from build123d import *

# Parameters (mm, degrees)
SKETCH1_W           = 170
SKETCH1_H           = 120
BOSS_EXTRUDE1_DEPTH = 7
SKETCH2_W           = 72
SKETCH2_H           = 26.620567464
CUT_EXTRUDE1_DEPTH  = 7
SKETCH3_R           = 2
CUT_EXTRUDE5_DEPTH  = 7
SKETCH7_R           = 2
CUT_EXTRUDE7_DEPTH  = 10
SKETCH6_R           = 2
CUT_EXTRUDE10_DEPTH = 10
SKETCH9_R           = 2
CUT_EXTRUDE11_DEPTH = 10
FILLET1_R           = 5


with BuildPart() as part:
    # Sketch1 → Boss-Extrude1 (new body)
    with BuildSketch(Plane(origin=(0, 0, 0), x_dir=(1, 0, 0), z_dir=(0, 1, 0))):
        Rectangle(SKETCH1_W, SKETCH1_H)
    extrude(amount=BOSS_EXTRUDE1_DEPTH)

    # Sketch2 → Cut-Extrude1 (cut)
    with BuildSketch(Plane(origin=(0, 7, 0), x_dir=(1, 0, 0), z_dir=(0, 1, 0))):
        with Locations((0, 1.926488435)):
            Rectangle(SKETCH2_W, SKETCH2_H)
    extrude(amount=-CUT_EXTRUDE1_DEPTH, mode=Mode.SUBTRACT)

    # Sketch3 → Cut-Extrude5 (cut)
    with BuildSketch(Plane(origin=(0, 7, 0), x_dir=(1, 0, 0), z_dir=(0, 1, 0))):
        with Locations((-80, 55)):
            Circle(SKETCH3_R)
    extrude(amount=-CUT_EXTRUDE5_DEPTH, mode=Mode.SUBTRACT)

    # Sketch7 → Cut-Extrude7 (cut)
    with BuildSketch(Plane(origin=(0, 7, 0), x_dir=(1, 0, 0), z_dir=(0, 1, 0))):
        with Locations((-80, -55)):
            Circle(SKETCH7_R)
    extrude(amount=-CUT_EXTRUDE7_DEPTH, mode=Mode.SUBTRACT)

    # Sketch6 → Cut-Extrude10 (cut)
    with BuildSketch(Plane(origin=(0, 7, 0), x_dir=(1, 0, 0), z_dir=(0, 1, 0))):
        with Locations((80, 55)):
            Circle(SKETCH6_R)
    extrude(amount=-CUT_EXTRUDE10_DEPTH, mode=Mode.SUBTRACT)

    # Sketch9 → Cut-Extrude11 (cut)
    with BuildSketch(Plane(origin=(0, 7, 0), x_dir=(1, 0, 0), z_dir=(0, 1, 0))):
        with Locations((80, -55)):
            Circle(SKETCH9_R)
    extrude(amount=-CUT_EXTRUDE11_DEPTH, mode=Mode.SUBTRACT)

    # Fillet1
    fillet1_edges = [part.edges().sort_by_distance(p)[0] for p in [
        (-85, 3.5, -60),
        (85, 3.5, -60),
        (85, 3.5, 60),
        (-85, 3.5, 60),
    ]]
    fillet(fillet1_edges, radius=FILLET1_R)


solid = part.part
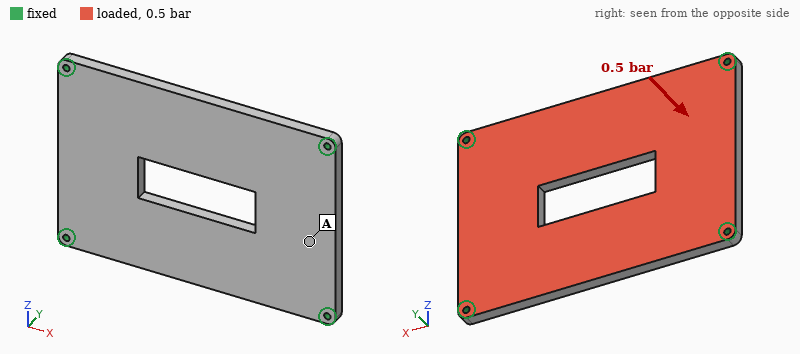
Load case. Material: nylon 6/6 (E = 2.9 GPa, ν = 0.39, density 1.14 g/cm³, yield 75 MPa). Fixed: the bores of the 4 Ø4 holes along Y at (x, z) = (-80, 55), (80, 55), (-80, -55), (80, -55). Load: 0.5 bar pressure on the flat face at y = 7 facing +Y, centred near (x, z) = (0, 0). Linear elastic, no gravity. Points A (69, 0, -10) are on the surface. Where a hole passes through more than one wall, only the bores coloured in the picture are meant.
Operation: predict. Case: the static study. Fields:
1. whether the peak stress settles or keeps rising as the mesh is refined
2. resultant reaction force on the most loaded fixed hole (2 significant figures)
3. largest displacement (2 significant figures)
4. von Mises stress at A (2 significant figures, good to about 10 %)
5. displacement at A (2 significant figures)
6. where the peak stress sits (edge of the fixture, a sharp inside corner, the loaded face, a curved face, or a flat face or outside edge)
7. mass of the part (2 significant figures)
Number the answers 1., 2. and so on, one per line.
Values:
1. keeps rising
2. 230 N
3. 2.5 mm
4. 5.6 MPa
5. 0.81 mm
6. edge of the fixture
7. 150 g
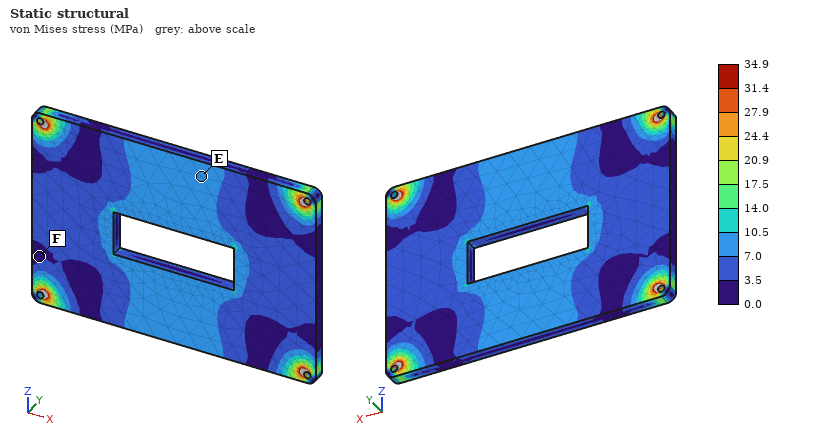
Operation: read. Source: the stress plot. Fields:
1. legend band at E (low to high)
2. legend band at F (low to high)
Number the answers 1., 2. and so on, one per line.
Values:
1. 7.0 to 10.5 MPa
2. 0.0 to 3.5 MPa
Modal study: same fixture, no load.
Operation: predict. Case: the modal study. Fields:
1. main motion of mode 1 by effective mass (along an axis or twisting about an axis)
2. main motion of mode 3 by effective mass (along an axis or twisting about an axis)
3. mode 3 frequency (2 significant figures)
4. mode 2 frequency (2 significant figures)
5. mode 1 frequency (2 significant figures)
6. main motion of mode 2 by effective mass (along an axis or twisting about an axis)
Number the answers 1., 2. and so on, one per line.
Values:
1. along Y
2. twisting about Z
3. 750 Hz
4. 500 Hz
5. 320 Hz
6. twisting about X
